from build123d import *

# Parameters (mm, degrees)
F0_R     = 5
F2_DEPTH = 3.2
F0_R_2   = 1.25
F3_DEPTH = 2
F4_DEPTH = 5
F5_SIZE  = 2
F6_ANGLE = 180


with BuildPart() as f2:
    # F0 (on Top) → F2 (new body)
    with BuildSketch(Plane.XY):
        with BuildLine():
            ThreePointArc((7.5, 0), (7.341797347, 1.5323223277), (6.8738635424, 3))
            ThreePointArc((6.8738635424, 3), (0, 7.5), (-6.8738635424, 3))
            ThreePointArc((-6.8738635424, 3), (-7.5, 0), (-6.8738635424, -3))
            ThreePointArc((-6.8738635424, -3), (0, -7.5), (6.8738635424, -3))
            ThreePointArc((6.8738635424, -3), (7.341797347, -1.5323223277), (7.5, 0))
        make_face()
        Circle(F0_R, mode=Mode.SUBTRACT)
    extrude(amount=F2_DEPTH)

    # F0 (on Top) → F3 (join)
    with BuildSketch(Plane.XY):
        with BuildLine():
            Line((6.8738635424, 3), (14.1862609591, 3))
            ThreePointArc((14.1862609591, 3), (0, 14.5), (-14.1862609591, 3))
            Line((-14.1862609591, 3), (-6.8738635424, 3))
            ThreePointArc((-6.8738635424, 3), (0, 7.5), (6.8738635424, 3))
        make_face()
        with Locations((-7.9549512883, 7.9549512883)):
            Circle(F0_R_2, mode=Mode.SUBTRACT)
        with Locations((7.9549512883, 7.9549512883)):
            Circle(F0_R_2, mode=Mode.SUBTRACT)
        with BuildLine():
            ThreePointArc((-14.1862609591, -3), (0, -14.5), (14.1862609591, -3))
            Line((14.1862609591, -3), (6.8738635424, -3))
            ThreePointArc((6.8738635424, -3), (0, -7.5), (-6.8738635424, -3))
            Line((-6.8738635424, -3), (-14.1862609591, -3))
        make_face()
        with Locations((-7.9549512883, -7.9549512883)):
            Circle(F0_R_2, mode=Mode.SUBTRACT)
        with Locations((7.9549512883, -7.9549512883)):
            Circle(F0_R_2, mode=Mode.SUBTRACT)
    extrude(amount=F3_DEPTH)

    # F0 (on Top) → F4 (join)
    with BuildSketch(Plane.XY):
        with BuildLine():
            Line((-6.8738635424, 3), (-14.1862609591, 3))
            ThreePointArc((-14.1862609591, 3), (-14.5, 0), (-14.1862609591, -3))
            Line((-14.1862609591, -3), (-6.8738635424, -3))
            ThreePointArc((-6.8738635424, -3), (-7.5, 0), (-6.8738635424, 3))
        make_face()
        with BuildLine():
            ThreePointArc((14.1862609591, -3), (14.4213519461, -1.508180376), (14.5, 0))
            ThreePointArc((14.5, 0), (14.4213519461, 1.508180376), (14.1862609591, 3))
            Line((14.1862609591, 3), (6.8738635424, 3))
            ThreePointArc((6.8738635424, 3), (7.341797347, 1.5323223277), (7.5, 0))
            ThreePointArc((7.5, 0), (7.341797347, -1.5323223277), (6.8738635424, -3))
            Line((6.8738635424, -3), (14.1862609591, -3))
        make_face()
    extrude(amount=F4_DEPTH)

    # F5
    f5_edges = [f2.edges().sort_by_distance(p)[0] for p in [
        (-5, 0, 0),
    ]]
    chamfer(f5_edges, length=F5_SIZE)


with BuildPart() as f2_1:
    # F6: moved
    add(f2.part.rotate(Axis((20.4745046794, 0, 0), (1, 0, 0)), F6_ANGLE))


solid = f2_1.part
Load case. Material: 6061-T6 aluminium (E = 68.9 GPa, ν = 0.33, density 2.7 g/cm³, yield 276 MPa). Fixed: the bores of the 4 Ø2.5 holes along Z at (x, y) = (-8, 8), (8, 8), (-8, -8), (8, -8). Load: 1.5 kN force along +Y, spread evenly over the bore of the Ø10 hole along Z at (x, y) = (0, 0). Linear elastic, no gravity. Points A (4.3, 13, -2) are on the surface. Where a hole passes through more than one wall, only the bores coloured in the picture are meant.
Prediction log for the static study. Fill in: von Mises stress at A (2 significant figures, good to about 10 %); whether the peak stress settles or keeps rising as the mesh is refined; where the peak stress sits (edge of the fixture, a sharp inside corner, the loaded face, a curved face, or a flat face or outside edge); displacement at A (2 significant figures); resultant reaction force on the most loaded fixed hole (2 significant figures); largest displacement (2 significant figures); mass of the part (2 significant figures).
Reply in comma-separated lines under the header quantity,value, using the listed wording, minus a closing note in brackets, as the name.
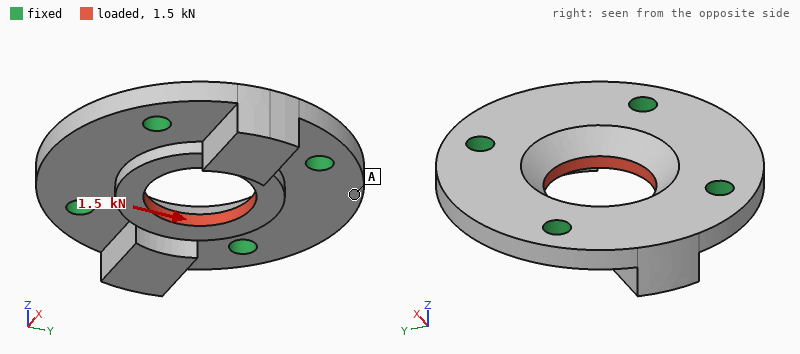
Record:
quantity,value
von Mises stress at A,11 MPa
whether the peak stress settles or keeps rising as the mesh is refined,keeps rising
where the peak stress sits,edge of the fixture
displacement at A,3.8 µm
resultant reaction force on the most loaded fixed hole,380 N
largest displacement,11 µm
mass of the part,3.9 g
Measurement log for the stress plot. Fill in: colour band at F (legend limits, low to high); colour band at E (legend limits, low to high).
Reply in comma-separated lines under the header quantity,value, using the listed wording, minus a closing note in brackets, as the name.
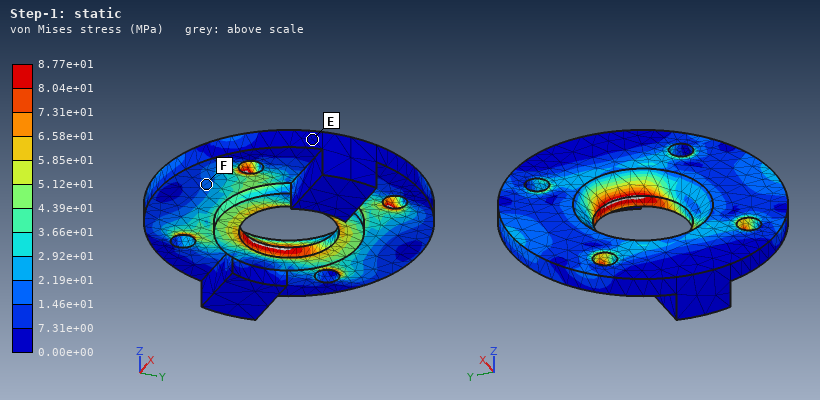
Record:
quantity,value
colour band at F,1.46e+01 to 2.19e+01 MPa
colour band at E,0.00e+00 to 7.31e+00 MPa
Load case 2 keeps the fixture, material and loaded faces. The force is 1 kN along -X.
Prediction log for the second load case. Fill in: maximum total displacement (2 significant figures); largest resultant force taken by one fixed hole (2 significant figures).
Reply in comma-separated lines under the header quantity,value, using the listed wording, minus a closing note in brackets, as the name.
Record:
quantity,value
maximum total displacement,6.9 µm
largest resultant force taken by one fixed hole,260 N
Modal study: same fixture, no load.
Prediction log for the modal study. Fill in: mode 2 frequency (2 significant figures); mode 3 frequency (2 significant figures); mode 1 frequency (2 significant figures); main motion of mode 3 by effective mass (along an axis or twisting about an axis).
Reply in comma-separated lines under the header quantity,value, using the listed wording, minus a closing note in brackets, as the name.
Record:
quantity,value
mode 2 frequency,26 kHz
mode 3 frequency,32 kHz
mode 1 frequency,25 kHz
main motion of mode 3 by effective mass,twisting about X
